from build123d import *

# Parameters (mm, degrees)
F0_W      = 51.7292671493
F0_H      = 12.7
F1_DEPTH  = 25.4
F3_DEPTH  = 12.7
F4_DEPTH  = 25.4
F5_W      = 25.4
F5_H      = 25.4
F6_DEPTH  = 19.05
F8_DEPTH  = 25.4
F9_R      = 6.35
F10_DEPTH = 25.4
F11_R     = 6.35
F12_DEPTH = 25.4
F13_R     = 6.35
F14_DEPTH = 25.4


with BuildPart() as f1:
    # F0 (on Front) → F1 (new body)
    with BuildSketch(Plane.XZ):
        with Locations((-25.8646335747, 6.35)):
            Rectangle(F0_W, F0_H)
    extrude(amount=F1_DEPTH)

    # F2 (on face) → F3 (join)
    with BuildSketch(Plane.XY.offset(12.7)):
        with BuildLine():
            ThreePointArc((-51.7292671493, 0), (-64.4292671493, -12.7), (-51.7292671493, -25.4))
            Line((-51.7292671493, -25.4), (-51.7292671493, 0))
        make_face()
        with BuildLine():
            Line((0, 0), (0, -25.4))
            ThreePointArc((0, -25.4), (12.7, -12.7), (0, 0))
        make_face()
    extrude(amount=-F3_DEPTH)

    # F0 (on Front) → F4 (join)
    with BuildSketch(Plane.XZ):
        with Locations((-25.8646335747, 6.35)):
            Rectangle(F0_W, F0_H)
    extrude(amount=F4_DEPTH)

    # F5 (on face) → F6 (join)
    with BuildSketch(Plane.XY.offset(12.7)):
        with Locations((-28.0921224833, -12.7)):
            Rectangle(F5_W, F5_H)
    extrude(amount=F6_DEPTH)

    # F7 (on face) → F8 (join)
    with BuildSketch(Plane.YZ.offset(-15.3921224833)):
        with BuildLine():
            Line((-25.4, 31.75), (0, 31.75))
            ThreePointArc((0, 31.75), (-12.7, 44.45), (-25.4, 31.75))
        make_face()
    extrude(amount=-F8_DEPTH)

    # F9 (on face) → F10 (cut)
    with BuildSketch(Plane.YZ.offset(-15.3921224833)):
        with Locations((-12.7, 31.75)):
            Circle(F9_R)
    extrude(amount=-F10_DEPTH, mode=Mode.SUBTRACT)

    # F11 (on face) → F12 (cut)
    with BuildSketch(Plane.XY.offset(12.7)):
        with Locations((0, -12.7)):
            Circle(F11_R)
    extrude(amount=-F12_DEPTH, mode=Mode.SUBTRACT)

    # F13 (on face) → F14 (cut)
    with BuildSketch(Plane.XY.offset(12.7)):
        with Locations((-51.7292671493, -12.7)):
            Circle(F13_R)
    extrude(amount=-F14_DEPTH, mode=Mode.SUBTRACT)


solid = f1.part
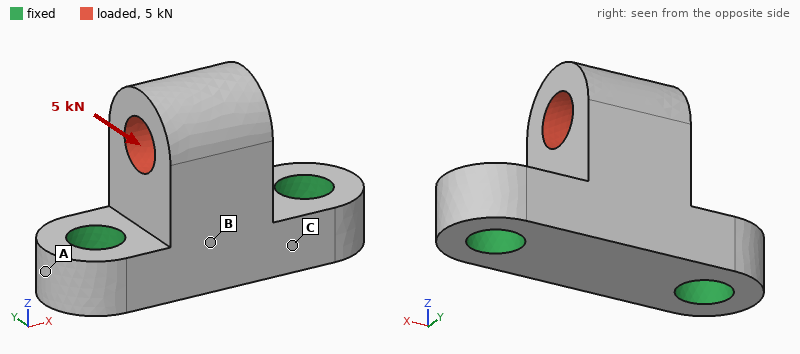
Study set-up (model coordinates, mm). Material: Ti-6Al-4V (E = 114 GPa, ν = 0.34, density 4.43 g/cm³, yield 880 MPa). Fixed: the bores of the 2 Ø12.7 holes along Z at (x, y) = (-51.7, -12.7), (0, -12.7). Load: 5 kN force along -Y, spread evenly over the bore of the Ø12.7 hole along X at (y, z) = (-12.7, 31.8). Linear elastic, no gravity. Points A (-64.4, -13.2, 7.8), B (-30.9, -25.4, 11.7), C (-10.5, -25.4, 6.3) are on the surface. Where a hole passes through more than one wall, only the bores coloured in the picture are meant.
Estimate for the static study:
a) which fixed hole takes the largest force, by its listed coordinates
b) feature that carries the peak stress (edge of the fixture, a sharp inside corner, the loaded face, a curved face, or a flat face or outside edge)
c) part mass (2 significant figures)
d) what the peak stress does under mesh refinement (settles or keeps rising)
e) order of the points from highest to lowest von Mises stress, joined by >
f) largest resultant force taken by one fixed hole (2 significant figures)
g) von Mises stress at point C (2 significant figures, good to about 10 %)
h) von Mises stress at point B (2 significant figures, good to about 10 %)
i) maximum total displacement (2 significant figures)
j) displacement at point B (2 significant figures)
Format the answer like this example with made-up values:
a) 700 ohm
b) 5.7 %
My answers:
a) (-51.7, -12.7)
b) edge of the fixture
c) 160 g
d) keeps rising
e) C > B > A
f) 2.9 kN
g) 71 MPa
h) 23 MPa
i) 68 µm
j) 20 µm
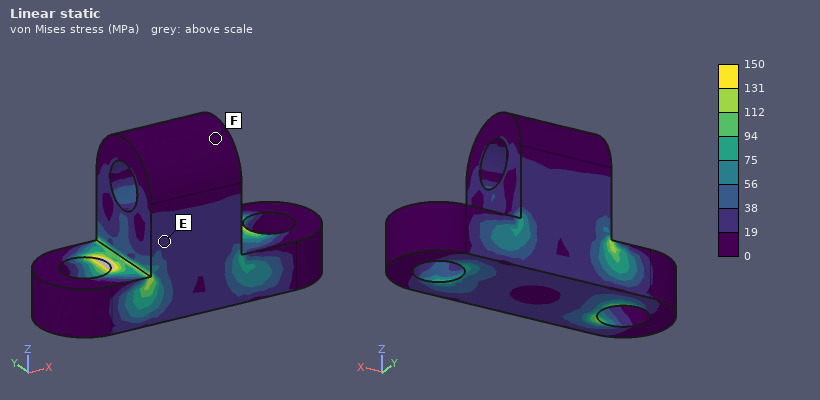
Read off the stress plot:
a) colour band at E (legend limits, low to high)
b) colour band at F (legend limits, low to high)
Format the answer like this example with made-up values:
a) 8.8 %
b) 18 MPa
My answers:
a) 19 to 38 MPa
b) 0 to 19 MPa
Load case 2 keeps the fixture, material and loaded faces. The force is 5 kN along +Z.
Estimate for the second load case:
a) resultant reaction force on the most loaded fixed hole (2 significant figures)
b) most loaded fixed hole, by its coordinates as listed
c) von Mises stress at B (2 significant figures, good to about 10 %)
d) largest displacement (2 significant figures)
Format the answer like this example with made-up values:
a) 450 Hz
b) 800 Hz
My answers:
a) 2.9 kN
b) (-51.7, -12.7)
c) 4.9 MPa
d) 7.7 µm
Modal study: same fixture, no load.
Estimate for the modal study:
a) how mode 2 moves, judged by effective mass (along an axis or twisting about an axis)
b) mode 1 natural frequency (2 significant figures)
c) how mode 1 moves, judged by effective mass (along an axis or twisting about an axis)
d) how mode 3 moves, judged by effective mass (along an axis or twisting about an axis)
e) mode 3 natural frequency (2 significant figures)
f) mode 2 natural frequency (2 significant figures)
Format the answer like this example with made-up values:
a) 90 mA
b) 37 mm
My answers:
a) along X
b) 6900 Hz
c) along Y
d) along Z
e) 17 kHz
f) 12 kHz
